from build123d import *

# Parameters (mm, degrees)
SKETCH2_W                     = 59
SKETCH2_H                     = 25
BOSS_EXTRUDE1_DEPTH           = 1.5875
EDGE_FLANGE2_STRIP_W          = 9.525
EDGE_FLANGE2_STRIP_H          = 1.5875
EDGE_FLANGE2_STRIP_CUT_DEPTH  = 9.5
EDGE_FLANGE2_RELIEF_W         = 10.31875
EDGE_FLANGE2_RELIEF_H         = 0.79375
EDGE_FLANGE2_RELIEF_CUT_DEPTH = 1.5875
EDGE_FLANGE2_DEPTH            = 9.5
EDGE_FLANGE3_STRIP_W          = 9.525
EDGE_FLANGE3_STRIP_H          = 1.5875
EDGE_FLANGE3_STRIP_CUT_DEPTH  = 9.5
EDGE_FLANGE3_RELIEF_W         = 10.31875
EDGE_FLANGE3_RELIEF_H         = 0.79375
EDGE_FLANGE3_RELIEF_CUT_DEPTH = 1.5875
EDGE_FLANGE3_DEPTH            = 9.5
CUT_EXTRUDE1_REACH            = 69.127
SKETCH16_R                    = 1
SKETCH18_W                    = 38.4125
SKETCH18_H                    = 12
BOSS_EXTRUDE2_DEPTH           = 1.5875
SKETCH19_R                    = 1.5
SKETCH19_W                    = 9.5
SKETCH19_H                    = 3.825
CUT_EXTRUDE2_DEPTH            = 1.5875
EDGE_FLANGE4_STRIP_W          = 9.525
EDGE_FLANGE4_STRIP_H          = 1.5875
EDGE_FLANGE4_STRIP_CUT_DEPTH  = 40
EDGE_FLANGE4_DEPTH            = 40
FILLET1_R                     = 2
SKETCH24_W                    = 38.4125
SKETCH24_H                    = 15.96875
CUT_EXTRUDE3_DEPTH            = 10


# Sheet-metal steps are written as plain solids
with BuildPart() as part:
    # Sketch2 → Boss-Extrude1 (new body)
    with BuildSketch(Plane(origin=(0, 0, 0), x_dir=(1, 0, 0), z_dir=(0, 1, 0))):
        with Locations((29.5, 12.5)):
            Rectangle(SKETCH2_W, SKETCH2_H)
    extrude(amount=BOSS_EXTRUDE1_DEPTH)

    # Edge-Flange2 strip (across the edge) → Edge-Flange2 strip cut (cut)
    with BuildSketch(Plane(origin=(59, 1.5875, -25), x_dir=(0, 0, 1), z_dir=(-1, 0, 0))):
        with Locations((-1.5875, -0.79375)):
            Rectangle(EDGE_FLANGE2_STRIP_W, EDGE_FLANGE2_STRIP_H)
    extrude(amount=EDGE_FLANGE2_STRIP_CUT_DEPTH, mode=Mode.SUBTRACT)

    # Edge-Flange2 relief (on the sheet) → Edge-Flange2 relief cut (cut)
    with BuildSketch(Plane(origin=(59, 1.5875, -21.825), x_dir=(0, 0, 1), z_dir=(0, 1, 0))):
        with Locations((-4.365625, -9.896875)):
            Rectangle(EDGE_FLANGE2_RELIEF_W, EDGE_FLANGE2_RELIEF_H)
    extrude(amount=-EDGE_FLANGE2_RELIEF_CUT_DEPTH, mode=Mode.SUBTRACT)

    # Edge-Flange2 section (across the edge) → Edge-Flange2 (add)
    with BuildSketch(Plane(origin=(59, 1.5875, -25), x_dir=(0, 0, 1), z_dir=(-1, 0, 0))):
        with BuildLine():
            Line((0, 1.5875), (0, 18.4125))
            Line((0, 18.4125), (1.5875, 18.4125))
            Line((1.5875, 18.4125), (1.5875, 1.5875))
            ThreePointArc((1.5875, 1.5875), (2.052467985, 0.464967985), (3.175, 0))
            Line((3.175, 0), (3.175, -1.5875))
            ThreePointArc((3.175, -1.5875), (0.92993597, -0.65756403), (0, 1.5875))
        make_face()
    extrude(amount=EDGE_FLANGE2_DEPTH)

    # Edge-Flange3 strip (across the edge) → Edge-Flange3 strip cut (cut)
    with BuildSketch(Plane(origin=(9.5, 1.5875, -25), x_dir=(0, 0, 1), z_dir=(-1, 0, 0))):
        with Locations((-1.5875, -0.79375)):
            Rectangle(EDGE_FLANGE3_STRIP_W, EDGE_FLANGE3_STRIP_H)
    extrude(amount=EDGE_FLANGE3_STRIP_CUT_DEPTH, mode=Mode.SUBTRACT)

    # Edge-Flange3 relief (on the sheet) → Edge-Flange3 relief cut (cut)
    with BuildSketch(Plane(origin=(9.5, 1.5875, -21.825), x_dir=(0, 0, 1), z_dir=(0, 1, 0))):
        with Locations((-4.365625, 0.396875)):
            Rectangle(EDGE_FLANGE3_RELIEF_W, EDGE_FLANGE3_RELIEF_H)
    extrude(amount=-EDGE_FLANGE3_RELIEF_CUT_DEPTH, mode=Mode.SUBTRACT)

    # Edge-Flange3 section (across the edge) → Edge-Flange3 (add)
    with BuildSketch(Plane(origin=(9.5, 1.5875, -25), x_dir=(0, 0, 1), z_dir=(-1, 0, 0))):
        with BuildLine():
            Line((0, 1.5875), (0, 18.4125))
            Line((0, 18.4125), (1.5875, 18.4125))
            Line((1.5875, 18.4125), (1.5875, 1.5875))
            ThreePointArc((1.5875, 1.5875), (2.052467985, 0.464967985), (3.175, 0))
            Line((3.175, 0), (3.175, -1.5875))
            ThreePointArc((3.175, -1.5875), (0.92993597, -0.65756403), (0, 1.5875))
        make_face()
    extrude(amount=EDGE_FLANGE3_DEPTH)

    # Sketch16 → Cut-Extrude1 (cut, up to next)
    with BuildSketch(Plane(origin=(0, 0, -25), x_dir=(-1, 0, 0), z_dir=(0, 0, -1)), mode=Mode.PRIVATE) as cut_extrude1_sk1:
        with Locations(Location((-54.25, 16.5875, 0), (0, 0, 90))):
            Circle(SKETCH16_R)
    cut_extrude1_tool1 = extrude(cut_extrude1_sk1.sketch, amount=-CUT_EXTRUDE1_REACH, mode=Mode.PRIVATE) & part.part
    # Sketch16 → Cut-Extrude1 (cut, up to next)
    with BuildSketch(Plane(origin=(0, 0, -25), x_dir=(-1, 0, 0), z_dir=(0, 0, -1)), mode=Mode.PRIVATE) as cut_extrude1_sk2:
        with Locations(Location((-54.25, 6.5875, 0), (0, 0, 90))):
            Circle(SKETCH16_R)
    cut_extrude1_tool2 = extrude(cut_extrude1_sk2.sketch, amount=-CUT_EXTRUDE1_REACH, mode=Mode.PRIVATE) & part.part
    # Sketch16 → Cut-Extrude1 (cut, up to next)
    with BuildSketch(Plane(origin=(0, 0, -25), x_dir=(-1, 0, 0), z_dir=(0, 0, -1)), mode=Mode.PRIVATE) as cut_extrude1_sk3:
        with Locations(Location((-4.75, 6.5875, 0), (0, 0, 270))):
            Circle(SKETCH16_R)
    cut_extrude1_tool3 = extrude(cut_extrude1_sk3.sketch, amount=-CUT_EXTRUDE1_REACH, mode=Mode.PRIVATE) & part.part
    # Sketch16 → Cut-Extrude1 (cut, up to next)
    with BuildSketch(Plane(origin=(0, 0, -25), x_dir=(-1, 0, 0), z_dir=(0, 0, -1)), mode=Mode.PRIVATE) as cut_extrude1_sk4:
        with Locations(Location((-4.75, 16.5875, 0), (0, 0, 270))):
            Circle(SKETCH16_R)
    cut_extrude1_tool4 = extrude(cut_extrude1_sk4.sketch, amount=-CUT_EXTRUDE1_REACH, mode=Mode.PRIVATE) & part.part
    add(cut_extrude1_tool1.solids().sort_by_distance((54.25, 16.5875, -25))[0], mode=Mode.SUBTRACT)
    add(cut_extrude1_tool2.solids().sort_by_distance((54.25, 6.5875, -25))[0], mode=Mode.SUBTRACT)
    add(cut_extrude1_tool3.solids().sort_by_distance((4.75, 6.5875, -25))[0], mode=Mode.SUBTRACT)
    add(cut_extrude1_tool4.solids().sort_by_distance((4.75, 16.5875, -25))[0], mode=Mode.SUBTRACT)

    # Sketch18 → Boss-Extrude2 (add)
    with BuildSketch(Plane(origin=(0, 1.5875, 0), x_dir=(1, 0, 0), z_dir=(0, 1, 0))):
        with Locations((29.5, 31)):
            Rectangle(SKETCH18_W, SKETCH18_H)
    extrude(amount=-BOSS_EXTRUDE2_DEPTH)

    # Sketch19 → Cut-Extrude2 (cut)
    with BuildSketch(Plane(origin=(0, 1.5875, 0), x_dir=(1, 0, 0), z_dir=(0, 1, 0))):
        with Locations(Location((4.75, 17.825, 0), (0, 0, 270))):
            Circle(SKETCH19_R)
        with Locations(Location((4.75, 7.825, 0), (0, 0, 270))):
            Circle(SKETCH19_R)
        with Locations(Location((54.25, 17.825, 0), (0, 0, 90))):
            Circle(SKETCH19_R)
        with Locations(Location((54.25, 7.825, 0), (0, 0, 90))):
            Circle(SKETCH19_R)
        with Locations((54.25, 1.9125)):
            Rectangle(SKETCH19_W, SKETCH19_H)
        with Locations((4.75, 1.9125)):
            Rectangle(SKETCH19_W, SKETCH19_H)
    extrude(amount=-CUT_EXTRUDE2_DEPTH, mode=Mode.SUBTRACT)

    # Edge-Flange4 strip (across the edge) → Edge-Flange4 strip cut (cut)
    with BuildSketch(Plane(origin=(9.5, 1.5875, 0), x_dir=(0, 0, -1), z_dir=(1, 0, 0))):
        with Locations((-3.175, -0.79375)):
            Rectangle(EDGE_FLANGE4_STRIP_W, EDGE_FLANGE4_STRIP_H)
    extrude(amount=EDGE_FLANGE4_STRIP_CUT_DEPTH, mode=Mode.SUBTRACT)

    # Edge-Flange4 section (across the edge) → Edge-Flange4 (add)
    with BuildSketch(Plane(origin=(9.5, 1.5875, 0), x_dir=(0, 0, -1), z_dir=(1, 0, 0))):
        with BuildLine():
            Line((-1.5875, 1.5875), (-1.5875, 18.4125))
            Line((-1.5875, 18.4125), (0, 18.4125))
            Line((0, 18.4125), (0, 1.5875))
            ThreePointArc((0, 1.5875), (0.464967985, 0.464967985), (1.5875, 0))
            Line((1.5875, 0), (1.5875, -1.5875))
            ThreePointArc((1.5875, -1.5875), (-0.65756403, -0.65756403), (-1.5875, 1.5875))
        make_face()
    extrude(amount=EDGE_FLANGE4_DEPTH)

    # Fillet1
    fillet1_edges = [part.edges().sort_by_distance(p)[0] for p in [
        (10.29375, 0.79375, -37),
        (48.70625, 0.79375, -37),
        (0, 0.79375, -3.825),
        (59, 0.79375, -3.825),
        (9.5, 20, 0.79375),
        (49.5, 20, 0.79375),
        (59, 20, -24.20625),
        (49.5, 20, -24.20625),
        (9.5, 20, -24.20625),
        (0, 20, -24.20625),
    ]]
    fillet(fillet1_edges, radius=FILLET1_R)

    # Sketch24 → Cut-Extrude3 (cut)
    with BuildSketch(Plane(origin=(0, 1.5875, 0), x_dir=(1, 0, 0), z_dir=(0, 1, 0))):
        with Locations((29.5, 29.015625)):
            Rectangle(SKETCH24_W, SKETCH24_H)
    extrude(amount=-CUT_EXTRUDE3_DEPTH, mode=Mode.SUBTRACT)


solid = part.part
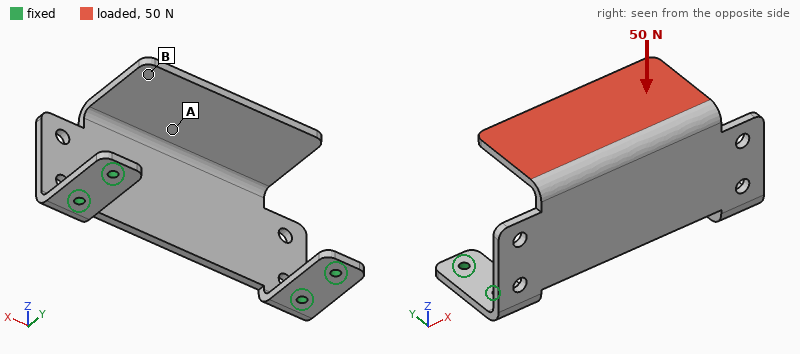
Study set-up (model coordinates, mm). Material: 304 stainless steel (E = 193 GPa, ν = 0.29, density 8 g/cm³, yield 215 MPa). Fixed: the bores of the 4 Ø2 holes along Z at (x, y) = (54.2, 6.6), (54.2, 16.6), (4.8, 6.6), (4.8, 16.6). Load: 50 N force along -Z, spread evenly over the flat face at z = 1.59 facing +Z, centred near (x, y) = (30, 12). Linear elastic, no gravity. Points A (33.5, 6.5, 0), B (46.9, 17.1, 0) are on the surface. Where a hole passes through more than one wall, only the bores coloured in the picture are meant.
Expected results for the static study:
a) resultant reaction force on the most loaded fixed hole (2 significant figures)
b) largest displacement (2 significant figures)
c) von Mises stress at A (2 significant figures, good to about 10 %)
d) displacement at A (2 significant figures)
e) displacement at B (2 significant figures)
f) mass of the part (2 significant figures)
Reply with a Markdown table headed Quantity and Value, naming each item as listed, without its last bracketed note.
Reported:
| Quantity | Value |
|---|---|
| resultant reaction force on the most loaded fixed hole | 27 N |
| largest displacement | 0.22 mm |
| von Mises stress at A | 15 MPa |
| displacement at A | 0.14 mm |
| displacement at B | 0.19 mm |
| mass of the part | 29 g |
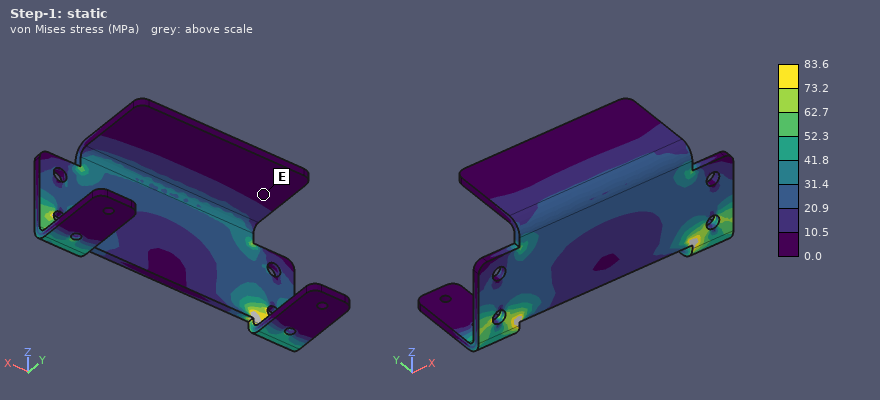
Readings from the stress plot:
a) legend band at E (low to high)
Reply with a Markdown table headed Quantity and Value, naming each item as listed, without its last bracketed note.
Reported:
| Quantity | Value |
|---|---|
| legend band at E | 0.0 to 10.5 MPa |
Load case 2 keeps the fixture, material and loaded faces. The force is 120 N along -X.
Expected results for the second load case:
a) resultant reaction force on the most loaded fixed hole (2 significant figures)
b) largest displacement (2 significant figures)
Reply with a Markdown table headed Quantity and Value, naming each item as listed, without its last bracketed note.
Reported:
| Quantity | Value |
|---|---|
| resultant reaction force on the most loaded fixed hole | 110 N |
| largest displacement | 0.13 mm |
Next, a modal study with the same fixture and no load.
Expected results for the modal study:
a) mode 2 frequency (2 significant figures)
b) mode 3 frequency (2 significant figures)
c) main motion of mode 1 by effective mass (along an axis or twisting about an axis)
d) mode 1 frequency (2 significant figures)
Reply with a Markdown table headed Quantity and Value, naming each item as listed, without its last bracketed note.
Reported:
| Quantity | Value |
|---|---|
| mode 2 frequency | 1500 Hz |
| mode 3 frequency | 1900 Hz |
| main motion of mode 1 by effective mass | along Y |
| mode 1 frequency | 510 Hz |
